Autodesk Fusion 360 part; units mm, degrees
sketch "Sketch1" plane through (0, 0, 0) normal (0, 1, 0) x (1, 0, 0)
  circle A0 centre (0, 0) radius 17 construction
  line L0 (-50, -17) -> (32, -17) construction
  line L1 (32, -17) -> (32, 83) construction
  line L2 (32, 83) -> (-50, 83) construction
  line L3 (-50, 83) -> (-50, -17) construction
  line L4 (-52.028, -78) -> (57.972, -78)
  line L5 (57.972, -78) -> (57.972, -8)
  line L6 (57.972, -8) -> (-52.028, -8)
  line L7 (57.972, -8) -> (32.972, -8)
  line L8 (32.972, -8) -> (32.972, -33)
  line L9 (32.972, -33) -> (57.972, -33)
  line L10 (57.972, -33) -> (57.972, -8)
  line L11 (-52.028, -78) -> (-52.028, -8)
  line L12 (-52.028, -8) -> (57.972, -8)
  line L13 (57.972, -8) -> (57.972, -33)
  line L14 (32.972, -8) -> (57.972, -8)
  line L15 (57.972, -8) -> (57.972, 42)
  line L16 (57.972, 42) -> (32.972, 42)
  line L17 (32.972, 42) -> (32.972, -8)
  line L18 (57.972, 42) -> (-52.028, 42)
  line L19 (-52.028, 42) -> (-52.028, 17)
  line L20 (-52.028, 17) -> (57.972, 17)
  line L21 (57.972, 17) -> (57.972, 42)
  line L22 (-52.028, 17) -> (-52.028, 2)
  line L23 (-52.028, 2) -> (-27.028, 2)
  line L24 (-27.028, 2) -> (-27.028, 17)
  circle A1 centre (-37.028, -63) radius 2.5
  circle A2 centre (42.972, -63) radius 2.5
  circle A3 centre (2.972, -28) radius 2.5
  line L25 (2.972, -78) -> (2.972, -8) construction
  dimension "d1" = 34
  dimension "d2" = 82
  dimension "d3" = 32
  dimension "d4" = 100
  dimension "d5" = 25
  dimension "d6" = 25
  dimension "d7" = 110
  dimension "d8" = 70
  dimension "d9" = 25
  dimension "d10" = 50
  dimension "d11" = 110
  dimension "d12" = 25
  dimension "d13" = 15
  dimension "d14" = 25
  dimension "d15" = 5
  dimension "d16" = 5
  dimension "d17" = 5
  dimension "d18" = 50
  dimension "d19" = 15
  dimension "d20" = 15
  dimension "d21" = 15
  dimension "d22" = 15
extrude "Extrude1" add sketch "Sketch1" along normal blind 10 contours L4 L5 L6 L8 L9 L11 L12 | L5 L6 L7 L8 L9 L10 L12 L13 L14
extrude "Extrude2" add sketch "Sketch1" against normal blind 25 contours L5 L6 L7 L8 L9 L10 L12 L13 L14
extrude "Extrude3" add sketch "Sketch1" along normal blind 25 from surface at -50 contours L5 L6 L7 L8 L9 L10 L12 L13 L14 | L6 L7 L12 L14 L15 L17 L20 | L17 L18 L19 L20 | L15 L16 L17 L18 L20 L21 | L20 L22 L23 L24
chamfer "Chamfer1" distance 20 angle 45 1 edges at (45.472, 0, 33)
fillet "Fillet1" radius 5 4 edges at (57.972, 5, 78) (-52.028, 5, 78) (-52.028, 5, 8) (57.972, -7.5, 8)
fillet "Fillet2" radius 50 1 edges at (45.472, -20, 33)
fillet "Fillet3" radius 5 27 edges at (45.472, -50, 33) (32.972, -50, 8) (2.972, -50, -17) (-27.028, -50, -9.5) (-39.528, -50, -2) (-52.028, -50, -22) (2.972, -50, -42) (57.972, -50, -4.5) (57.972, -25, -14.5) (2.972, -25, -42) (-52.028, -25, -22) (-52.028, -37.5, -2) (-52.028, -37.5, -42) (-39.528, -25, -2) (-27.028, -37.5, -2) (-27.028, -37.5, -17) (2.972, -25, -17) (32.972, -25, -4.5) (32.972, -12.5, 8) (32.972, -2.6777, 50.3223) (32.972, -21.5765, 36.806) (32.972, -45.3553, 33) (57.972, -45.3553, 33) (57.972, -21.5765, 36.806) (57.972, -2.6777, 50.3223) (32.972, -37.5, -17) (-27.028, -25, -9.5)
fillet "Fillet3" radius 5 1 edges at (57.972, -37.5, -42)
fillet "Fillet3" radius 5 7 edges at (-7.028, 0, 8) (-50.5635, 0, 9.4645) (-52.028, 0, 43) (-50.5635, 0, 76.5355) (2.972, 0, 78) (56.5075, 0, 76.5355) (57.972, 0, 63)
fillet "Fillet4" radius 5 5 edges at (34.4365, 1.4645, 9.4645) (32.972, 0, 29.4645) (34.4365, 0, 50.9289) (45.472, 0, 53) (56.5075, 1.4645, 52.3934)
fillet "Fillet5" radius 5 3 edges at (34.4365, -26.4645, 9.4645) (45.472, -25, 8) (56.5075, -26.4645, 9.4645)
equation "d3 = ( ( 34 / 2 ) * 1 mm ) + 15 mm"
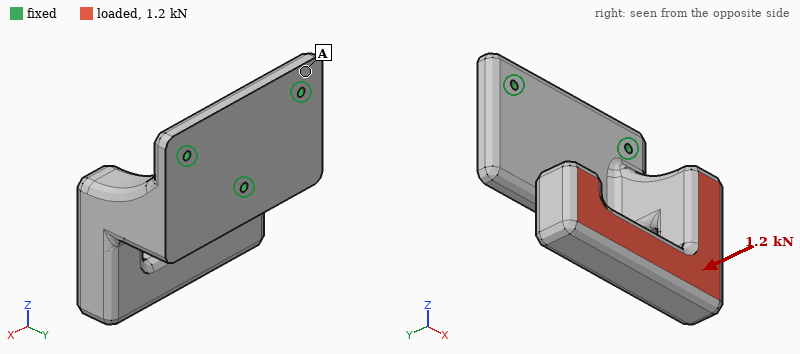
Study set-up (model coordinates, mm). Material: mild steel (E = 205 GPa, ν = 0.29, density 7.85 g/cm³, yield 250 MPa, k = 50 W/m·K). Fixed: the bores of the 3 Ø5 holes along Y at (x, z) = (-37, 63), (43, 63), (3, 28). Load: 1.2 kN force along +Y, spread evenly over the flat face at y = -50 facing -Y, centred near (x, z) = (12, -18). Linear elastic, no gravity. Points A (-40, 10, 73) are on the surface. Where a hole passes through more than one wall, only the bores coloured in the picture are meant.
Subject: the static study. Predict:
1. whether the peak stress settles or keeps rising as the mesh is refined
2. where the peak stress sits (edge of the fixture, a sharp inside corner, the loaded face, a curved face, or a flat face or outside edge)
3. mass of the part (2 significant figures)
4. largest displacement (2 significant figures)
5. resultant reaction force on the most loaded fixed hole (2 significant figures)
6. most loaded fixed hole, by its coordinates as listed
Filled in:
keeps rising
edge of the fixture
1.6 kg
0.13 mm
2.1 kN
(3, 28)
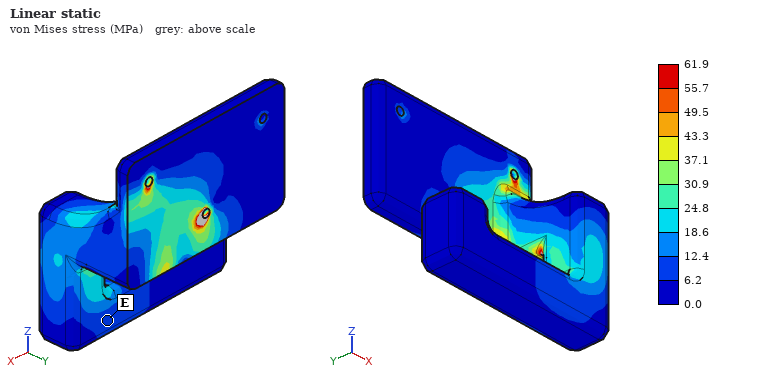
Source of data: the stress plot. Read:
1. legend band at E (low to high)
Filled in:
6.2 to 12.4 MPa
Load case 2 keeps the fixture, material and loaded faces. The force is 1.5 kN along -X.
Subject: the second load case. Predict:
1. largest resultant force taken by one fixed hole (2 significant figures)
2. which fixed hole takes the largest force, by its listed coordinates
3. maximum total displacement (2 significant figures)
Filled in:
2.2 kN
(3, 28)
0.15 mm
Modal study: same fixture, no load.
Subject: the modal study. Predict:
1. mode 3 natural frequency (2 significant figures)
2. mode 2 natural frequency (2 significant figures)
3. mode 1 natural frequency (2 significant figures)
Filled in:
1100 Hz
660 Hz
560 Hz
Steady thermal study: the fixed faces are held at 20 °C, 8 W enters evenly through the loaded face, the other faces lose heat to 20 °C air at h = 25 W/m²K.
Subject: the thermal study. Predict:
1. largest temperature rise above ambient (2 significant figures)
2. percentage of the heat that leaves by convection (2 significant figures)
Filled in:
14 K
58 %
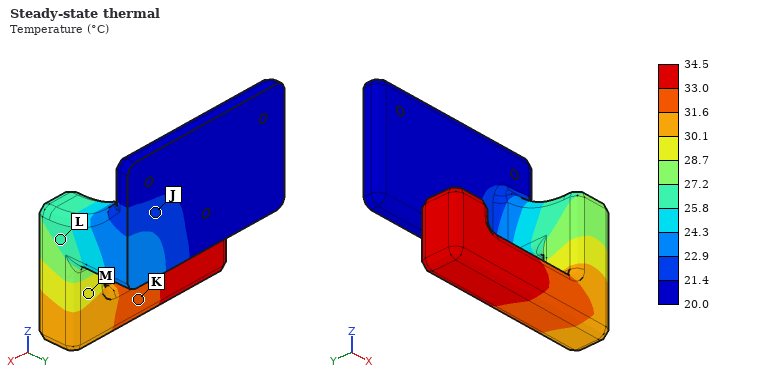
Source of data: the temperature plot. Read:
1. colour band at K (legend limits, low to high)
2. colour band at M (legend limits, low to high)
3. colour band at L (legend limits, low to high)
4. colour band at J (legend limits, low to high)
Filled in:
31.6 to 33.0 °C
28.7 to 30.1 °C
25.8 to 27.2 °C
21.4 to 22.9 °C
